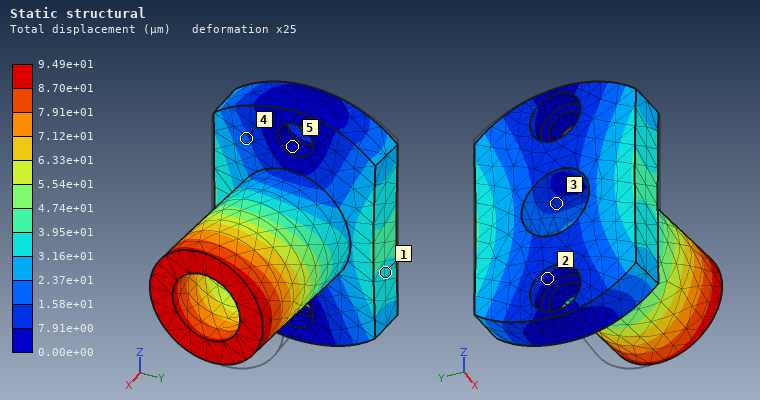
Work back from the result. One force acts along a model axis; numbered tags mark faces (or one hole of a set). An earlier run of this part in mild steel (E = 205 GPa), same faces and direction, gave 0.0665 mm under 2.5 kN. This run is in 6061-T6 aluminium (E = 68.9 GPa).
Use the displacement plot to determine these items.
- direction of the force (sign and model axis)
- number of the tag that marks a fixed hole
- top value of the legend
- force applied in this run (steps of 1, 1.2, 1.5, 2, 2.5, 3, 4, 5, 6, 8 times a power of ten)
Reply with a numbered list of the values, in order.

1. -Y
2. 5
3. 9.49e+01 µm
4. 1.2 kN
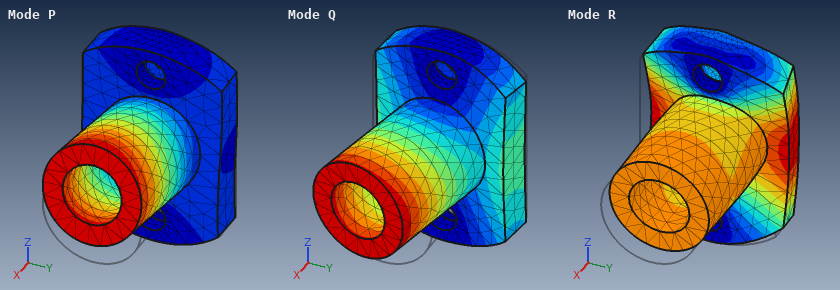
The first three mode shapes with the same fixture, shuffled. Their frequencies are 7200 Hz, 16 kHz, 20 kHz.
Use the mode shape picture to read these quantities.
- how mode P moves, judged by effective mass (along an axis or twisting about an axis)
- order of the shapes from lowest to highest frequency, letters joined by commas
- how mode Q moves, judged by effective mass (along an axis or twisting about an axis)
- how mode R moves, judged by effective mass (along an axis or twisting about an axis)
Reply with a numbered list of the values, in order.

1. along Z
2. Q, P, R
3. along Y
4. along X
